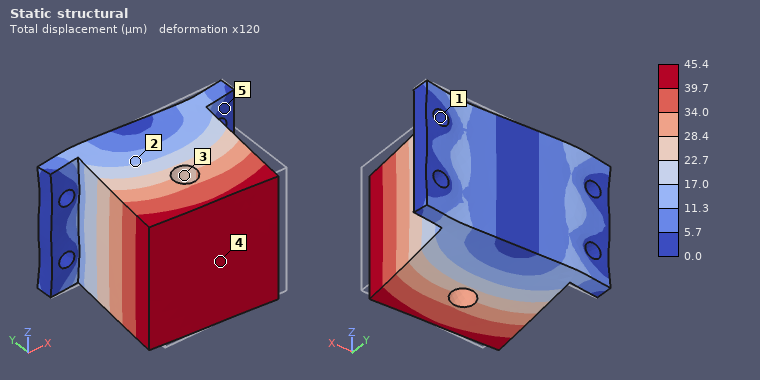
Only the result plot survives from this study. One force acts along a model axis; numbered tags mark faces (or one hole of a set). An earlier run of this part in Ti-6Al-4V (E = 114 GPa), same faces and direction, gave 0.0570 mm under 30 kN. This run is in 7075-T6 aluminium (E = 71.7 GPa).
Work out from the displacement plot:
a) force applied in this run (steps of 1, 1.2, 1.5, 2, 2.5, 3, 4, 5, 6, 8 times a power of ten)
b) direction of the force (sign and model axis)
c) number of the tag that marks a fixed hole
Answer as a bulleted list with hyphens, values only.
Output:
- 15 kN
- -X
- 1
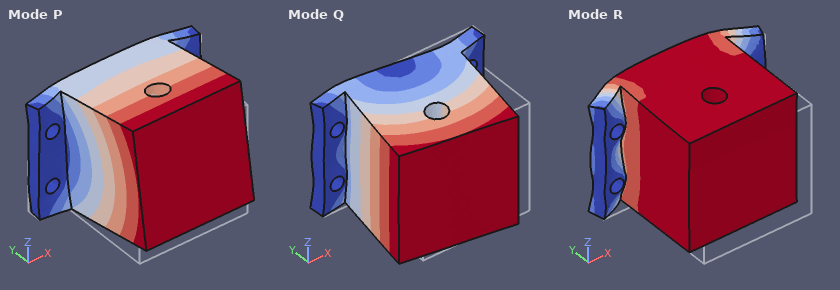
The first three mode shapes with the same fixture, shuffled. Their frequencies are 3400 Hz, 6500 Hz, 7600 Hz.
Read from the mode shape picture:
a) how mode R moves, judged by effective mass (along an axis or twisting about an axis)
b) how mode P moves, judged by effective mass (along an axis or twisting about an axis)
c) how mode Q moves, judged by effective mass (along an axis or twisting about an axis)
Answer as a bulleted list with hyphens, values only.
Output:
- along Y
- along Z
- along X
